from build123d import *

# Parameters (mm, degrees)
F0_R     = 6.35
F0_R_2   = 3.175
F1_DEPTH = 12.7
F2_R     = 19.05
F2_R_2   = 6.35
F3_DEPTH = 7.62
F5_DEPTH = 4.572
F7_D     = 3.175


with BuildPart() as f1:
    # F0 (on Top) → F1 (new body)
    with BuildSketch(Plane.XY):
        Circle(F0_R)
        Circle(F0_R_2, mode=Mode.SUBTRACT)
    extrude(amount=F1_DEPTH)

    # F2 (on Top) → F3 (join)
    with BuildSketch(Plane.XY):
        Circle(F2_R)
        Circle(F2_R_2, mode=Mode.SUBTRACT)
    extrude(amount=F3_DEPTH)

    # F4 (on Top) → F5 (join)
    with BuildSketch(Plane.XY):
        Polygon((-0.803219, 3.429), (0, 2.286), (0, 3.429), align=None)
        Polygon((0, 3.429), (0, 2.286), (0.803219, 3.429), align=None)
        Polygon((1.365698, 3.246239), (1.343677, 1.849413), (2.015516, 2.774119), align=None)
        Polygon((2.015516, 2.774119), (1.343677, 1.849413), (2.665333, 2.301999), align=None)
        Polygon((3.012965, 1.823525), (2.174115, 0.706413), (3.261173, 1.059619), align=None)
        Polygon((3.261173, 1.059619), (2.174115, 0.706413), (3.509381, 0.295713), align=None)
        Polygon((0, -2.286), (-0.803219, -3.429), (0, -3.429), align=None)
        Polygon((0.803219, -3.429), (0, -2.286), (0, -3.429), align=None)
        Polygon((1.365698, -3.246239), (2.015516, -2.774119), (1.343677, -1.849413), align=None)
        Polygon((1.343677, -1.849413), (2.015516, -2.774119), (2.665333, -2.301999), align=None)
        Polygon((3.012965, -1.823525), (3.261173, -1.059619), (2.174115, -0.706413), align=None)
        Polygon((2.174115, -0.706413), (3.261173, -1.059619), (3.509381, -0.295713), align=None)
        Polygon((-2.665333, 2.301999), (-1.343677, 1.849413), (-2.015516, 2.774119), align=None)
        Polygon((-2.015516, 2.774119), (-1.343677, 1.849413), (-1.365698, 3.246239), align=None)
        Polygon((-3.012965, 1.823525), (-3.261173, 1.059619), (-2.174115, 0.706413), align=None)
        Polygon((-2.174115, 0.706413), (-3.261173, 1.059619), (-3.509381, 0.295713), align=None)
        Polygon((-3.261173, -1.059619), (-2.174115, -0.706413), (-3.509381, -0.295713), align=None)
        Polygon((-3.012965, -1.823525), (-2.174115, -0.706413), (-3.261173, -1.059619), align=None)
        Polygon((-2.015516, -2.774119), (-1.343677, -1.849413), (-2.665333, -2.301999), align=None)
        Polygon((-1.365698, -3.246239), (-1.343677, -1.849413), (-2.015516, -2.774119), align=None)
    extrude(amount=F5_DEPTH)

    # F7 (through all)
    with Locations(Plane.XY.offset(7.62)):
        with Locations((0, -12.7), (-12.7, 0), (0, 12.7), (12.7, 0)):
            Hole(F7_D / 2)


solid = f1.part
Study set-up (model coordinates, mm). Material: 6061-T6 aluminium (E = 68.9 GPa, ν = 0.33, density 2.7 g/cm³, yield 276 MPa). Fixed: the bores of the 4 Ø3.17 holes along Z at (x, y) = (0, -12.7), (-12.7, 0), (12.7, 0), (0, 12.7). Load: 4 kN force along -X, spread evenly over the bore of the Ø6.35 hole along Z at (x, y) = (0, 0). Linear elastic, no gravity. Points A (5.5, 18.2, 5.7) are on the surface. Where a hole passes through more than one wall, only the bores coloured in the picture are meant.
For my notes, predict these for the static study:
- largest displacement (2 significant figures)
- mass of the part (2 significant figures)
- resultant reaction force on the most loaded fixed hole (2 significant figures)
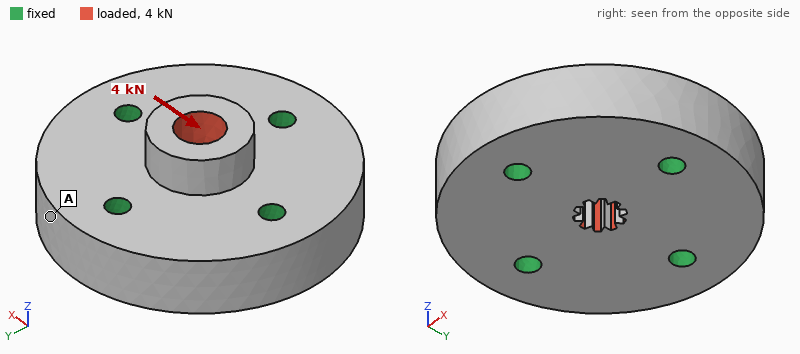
11 µm
24 g
1.4 kN
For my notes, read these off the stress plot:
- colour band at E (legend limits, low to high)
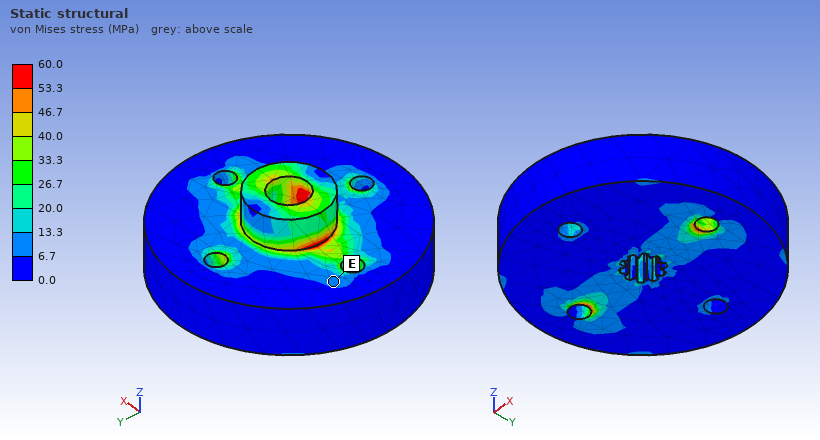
6.7 to 13.3 MPa
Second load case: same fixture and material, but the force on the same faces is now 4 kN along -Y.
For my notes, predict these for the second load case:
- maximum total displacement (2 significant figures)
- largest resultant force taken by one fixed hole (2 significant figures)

11 µm
1.4 kN
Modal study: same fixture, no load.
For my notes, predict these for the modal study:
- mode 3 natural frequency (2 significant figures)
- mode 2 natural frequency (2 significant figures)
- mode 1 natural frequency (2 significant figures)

45 kHz
45 kHz
43 kHz
